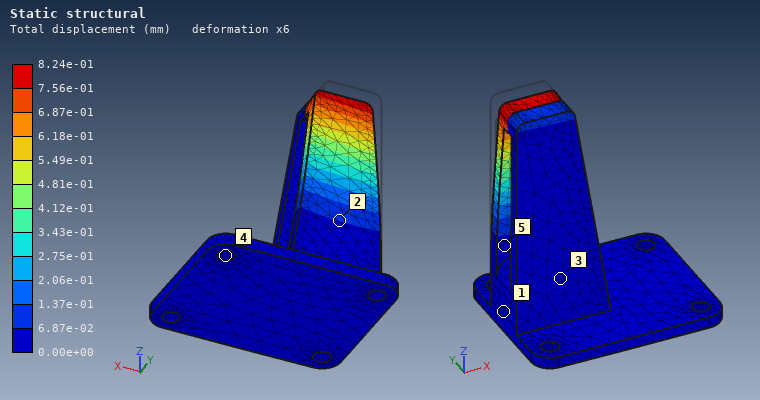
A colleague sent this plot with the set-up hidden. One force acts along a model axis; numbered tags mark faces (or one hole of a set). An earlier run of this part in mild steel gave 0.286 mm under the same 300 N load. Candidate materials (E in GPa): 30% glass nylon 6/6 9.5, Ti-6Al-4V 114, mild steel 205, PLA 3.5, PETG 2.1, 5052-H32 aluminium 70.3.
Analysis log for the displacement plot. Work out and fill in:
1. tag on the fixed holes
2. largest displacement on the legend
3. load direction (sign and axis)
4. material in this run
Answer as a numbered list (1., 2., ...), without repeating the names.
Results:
1. 4
2. 8.24e-01 mm
3. -Y
4. 5052-H32 aluminium
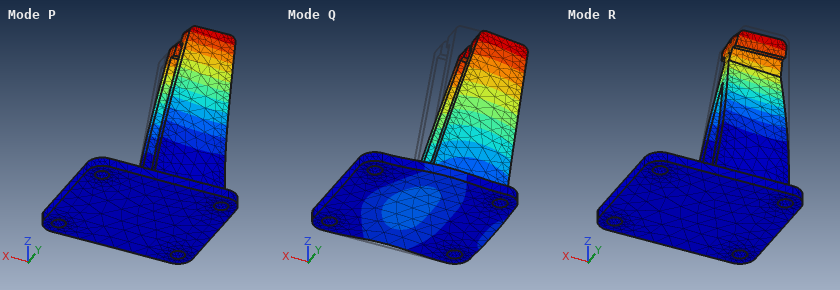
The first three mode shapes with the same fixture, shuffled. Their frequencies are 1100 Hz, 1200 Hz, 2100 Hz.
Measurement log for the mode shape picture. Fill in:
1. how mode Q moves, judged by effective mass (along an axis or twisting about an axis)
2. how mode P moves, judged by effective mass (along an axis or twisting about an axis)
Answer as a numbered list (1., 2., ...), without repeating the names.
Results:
1. along X
2. along Y
